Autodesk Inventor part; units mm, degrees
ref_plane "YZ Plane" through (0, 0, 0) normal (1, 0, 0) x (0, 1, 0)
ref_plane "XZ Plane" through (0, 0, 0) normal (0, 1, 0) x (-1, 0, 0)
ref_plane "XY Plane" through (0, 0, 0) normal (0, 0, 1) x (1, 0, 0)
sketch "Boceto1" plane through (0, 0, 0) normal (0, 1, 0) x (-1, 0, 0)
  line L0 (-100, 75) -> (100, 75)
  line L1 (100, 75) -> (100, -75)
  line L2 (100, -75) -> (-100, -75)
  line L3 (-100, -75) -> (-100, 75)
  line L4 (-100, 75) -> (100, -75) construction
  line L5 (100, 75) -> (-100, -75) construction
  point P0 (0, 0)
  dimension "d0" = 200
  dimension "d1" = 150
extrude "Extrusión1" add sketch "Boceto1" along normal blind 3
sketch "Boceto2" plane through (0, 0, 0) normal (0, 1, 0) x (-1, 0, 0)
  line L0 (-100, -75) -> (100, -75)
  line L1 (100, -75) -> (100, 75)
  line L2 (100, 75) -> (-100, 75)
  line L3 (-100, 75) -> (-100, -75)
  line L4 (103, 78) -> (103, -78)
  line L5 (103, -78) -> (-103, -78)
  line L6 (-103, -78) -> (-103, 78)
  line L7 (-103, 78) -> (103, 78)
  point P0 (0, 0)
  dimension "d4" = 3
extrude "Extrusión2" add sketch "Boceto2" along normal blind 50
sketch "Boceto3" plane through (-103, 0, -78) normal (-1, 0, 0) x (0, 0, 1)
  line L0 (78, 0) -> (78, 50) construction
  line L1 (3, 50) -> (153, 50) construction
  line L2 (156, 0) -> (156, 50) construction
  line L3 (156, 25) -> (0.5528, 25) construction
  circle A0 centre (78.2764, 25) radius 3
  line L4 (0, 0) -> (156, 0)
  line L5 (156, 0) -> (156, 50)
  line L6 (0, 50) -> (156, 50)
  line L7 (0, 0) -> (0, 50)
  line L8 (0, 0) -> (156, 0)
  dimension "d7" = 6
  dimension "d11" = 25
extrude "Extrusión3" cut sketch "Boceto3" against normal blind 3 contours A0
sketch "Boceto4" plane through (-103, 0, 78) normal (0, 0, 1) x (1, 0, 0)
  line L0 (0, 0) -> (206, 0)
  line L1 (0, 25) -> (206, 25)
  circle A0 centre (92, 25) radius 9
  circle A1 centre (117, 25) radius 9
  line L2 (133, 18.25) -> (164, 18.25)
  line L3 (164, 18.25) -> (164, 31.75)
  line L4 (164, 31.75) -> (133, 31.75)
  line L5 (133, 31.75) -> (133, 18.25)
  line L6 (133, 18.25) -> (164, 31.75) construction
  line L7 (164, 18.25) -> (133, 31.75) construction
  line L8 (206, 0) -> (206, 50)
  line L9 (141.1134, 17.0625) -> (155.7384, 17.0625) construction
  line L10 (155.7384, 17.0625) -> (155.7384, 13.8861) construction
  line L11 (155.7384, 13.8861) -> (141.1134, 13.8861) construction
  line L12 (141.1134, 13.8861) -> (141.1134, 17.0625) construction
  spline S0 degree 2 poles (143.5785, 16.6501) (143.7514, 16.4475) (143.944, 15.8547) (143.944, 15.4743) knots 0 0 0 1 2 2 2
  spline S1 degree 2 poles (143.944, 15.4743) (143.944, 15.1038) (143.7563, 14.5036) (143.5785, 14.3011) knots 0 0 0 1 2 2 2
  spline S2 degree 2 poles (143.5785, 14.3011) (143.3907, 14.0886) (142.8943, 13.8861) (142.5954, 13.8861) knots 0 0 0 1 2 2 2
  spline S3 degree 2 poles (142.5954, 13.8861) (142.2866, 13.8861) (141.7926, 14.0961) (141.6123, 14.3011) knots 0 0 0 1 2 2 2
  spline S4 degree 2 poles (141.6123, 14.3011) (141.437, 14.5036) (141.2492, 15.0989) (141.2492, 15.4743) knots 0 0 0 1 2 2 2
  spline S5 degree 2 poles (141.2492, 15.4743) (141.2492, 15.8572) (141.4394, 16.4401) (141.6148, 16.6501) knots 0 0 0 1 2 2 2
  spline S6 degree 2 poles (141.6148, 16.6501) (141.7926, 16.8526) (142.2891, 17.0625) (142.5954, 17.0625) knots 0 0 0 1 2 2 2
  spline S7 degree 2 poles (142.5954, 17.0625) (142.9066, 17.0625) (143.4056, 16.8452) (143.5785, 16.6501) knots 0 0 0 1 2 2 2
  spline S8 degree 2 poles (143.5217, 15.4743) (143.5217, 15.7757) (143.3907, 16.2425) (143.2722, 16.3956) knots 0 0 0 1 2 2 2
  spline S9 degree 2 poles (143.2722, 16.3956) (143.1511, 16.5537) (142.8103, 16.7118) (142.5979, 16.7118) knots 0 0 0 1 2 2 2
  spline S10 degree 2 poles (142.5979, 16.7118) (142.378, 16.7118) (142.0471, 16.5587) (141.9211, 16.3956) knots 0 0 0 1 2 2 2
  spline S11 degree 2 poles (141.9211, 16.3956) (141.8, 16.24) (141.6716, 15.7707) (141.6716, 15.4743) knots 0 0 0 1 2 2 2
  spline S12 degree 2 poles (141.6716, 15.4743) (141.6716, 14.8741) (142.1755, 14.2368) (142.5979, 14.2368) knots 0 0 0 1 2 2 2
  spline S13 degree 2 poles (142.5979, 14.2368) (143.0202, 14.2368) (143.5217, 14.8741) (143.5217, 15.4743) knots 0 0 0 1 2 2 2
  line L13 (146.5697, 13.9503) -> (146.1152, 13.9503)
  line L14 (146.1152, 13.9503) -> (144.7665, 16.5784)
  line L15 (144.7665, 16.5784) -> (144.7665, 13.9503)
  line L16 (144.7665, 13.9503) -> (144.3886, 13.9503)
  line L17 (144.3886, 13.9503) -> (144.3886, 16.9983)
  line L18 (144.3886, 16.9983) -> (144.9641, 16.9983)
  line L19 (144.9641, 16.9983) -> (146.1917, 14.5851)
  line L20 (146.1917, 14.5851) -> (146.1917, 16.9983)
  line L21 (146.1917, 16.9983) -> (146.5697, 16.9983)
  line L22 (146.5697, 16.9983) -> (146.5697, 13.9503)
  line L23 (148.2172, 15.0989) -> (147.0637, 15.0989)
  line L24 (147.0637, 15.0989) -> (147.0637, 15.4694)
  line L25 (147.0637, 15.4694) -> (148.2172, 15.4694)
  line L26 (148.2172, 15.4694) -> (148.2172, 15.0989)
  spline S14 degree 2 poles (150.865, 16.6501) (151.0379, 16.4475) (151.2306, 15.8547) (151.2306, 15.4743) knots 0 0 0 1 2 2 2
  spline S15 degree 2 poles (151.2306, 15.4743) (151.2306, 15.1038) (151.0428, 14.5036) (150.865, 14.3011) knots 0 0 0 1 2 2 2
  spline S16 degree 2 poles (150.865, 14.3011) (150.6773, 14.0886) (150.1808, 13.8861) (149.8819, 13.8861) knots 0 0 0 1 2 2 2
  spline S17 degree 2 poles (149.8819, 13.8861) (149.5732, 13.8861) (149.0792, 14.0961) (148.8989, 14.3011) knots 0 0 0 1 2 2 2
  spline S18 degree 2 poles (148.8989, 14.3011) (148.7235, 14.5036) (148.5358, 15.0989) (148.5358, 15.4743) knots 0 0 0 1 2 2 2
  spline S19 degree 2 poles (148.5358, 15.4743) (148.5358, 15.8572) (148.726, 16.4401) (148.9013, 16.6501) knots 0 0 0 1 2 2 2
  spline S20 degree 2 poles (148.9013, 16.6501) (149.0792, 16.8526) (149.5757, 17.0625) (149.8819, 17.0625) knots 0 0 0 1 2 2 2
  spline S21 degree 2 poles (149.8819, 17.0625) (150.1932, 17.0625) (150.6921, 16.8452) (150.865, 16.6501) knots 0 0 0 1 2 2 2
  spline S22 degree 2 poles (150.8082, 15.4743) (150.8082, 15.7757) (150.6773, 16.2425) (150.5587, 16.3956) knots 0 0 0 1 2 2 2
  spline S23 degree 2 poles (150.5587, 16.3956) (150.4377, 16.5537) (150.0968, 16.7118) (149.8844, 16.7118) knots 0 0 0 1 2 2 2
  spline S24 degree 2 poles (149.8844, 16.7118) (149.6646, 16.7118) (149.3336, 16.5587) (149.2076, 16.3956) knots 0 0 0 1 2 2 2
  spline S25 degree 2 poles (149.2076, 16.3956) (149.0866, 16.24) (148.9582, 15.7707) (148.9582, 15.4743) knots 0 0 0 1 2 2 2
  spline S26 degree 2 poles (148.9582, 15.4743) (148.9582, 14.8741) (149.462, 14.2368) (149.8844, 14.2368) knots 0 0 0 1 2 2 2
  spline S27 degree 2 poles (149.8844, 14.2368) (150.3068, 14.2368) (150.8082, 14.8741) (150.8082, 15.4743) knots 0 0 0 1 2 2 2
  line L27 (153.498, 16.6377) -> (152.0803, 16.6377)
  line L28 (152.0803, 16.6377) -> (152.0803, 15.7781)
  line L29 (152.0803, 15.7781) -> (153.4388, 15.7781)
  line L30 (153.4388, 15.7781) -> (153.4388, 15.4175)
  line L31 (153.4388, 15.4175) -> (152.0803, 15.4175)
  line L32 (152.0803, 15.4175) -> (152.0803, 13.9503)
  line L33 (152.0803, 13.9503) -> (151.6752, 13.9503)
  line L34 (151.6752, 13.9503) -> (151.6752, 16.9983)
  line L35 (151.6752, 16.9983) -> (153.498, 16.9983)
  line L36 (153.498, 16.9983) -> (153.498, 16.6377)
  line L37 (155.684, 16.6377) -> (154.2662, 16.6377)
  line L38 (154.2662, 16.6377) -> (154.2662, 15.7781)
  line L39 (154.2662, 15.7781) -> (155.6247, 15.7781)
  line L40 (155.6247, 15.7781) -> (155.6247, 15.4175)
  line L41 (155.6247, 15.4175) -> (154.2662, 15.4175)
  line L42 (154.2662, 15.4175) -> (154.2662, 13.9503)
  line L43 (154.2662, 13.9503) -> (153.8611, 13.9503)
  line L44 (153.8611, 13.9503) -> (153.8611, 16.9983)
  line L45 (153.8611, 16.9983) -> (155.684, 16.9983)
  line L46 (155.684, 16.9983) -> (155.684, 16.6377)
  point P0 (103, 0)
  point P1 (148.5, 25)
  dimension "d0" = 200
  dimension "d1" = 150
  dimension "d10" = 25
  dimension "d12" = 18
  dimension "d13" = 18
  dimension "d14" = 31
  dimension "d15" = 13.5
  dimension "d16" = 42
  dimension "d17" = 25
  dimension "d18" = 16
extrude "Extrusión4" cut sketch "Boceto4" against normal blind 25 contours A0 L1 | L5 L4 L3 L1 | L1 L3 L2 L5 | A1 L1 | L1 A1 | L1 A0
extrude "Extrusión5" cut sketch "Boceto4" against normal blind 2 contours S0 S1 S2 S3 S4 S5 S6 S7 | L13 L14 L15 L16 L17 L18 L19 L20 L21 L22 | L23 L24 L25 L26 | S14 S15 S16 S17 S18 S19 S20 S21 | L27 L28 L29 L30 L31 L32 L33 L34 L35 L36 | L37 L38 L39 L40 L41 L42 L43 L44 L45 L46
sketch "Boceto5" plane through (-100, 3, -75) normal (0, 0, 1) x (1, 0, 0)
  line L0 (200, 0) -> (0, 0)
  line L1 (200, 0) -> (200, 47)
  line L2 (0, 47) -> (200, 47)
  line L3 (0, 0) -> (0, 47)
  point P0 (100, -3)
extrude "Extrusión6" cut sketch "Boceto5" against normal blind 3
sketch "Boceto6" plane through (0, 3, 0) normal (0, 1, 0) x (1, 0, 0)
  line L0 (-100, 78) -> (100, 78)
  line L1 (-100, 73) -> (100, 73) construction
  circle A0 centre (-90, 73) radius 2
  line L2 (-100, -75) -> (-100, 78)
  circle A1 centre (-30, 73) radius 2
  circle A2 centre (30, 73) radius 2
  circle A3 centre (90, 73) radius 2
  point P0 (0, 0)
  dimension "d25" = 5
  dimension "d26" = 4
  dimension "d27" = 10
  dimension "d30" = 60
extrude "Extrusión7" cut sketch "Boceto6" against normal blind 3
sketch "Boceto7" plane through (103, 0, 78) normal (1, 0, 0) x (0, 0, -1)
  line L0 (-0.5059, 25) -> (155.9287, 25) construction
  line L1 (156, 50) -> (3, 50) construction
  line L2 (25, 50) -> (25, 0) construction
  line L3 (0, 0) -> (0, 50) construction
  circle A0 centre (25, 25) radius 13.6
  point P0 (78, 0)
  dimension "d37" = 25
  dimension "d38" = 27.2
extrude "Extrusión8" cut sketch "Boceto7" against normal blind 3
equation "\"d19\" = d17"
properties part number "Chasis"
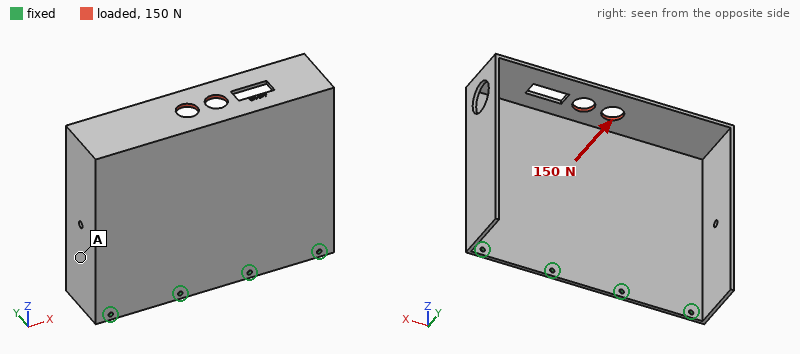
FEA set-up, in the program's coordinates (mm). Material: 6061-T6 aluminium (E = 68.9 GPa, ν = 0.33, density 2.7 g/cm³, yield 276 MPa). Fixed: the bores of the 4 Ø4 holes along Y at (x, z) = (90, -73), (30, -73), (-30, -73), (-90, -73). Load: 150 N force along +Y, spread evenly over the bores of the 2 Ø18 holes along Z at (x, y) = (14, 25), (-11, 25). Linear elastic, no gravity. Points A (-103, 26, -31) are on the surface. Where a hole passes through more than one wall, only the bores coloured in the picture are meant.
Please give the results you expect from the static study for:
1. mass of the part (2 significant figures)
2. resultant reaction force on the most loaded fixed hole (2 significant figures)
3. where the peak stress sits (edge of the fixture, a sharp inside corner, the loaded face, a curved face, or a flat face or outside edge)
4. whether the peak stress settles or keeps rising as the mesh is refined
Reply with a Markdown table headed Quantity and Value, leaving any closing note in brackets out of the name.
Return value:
| Quantity | Value |
|---|---|
| mass of the part | 440 g |
| resultant reaction force on the most loaded fixed hole | 89 N |
| where the peak stress sits | edge of the fixture |
| whether the peak stress settles or keeps rising as the mesh is refined | keeps rising |
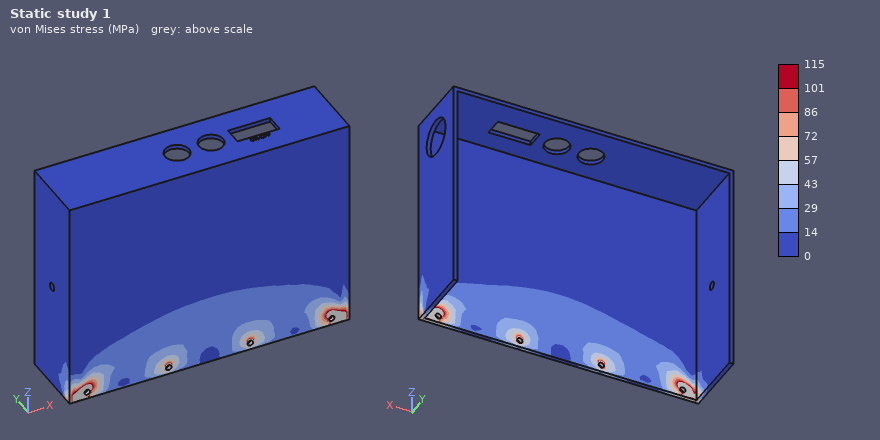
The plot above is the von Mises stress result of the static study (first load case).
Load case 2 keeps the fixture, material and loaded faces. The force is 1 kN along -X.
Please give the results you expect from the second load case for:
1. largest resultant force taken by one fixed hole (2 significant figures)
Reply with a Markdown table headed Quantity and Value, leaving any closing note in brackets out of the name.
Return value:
| Quantity | Value |
|---|---|
| largest resultant force taken by one fixed hole | 800 N |
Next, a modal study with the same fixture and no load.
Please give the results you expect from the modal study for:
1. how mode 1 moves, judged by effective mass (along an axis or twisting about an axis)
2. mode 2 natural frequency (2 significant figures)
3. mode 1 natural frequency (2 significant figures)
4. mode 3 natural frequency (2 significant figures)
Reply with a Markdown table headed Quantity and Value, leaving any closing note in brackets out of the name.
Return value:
| Quantity | Value |
|---|---|
| how mode 1 moves, judged by effective mass | along Y |
| mode 2 natural frequency | 160 Hz |
| mode 1 natural frequency | 99 Hz |
| mode 3 natural frequency | 650 Hz |
